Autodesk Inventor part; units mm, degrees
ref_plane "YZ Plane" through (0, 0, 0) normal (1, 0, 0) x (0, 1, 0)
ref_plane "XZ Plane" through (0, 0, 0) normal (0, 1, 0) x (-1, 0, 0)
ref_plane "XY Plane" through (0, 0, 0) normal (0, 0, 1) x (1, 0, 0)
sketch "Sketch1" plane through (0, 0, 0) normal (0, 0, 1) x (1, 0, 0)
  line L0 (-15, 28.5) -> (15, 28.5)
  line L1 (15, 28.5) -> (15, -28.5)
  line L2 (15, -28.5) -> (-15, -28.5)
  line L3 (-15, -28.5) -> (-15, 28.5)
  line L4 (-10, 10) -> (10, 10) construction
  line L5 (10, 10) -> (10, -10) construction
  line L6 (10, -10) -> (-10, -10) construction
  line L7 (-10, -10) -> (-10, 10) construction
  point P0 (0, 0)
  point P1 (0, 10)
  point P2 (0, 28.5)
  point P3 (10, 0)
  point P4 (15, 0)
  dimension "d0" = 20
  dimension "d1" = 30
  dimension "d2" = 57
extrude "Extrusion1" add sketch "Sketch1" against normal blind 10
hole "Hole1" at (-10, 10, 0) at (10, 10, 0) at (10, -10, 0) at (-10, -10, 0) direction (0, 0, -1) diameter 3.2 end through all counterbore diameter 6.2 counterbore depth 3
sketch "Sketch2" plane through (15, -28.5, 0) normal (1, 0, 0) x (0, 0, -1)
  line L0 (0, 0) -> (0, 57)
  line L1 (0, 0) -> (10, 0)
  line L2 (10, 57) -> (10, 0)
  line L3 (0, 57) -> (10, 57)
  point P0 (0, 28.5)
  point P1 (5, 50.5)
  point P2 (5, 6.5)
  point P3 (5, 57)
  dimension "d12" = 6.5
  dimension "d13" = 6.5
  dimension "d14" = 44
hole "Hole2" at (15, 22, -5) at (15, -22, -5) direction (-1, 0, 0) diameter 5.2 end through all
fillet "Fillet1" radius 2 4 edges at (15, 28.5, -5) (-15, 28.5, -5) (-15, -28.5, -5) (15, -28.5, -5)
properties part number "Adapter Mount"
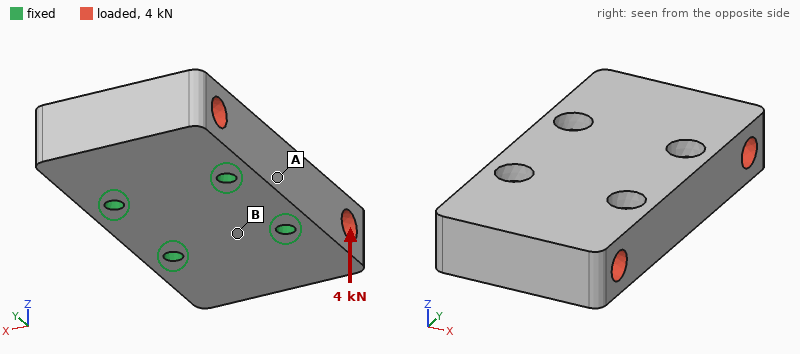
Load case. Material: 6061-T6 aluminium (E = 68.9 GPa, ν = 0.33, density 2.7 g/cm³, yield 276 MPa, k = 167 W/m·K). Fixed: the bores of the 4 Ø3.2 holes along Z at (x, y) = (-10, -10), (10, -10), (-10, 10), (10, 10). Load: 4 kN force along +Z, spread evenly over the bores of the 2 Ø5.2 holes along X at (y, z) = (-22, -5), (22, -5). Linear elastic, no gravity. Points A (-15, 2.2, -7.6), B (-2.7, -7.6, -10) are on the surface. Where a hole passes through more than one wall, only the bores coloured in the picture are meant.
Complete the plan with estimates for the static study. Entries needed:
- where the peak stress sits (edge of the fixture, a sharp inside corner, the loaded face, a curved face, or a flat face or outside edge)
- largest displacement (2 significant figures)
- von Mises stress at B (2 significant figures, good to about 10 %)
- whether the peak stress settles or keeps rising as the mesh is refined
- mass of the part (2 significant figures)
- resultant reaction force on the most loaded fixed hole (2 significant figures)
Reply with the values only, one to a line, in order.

edge of the fixture
32 µm
25 MPa
keeps rising
41 g
1.1 kN
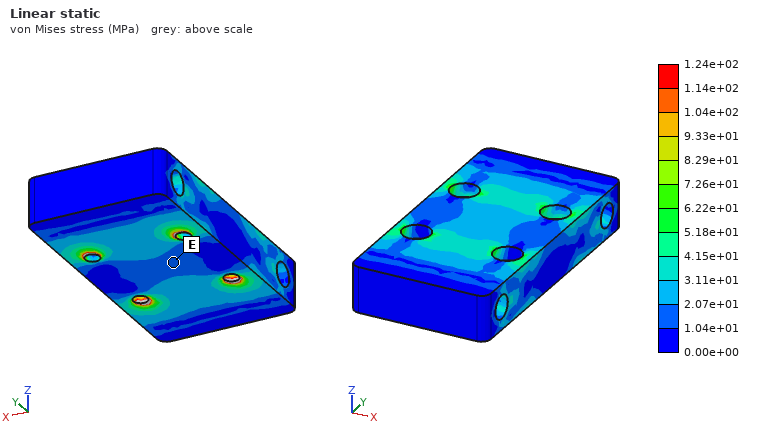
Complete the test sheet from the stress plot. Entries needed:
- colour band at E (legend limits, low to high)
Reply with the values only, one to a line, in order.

1.04e+01 to 2.07e+01 MPa
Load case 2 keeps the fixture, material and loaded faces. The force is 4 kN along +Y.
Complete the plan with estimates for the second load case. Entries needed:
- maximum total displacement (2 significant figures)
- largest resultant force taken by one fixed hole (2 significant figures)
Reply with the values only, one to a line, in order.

3.3 µm
1.0 kN
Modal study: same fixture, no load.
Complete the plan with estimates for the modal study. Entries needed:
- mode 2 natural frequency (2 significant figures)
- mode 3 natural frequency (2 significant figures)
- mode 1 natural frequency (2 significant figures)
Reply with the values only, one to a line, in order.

15 kHz
27 kHz
15 kHz
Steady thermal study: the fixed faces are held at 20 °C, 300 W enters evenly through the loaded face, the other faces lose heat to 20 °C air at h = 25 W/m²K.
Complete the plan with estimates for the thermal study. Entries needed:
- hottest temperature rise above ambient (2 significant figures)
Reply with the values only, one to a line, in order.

54 K
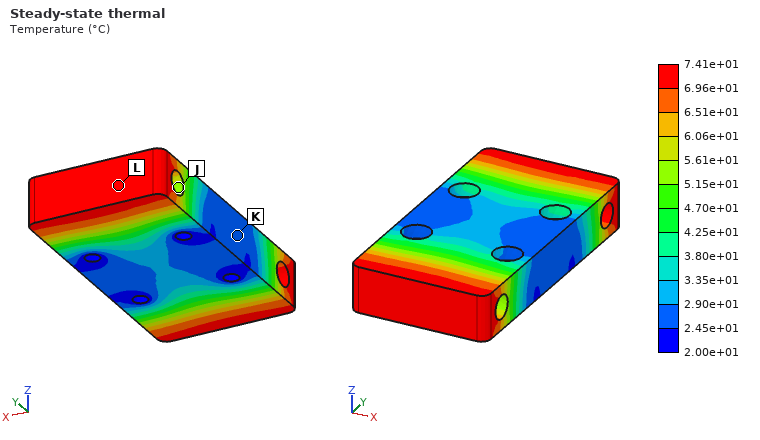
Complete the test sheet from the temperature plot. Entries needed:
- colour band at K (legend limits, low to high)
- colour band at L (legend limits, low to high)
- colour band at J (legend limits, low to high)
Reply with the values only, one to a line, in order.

2.45e+01 to 2.90e+01 °C
6.96e+01 to 7.41e+01 °C
5.15e+01 to 5.61e+01 °C
